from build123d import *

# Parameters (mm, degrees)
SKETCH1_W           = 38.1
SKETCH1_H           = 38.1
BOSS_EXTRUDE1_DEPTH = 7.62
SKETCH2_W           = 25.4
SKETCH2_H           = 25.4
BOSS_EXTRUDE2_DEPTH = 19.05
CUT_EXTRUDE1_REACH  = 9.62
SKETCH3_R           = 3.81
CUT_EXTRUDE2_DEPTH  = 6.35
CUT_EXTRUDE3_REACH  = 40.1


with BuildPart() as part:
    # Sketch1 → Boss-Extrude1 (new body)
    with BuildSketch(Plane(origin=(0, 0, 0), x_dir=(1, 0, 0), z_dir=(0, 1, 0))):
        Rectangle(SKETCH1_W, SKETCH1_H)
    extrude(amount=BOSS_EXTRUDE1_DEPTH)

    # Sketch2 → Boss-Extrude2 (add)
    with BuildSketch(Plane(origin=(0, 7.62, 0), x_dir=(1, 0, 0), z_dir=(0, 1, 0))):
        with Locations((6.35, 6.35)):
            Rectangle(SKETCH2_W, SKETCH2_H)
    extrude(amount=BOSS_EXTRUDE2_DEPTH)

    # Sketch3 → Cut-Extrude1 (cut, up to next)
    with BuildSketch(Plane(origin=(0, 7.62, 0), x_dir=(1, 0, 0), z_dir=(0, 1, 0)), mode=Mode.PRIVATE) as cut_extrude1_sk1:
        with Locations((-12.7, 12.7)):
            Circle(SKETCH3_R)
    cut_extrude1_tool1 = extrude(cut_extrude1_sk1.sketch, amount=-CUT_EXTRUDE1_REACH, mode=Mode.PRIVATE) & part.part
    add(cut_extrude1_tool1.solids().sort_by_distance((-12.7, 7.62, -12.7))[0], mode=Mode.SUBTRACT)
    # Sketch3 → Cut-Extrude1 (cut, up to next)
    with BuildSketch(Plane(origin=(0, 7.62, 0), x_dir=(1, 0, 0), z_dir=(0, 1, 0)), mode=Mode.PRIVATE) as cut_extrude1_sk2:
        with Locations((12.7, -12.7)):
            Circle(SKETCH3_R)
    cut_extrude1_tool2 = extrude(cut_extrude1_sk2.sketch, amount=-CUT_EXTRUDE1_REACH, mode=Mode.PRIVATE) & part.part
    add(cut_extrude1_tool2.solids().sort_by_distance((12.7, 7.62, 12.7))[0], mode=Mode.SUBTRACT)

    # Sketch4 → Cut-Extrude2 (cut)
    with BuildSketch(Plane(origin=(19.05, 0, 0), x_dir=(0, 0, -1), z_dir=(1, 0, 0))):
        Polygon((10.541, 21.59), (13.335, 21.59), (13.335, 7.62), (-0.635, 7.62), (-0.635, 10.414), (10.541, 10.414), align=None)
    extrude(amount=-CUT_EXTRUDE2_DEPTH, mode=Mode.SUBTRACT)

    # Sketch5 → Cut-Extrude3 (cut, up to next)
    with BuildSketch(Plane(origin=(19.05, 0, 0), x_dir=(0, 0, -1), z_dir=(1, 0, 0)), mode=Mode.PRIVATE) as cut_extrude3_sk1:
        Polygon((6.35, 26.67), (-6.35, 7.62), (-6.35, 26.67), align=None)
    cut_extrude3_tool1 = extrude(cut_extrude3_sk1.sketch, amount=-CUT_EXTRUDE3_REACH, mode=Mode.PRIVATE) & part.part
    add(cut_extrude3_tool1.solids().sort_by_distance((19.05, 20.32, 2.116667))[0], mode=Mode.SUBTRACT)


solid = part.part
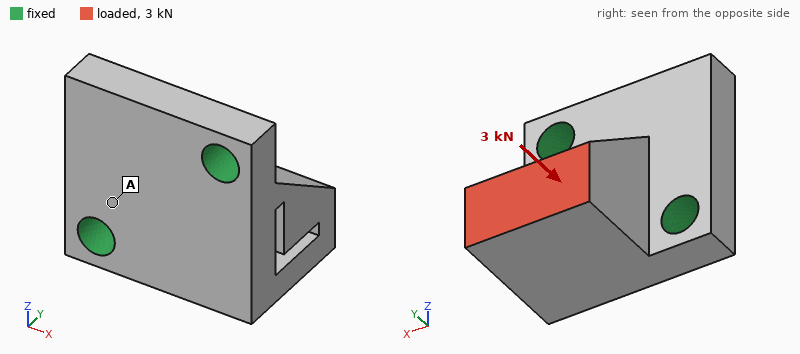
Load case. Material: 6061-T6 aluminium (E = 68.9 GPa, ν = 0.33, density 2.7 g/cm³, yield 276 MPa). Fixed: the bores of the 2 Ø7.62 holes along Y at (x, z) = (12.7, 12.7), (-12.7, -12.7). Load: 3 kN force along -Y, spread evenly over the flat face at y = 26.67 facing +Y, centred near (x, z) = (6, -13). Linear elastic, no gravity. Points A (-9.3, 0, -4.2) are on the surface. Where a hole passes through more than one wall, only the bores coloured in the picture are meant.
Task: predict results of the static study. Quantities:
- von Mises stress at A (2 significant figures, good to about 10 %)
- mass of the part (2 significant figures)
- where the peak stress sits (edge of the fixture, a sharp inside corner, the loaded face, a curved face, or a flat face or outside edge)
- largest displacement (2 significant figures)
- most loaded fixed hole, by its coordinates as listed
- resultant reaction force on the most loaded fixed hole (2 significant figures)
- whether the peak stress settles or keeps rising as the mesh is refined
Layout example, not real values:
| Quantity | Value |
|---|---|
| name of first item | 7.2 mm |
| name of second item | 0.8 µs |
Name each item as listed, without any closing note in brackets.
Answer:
| Quantity | Value |
|---|---|
| von Mises stress at A | 23 MPa |
| mass of the part | 52 g |
| where the peak stress sits | edge of the fixture |
| largest displacement | 73 µm |
| most loaded fixed hole, by its coordinates as listed | (-12.7, -12.7) |
| resultant reaction force on the most loaded fixed hole | 2.0 kN |
| whether the peak stress settles or keeps rising as the mesh is refined | keeps rising |
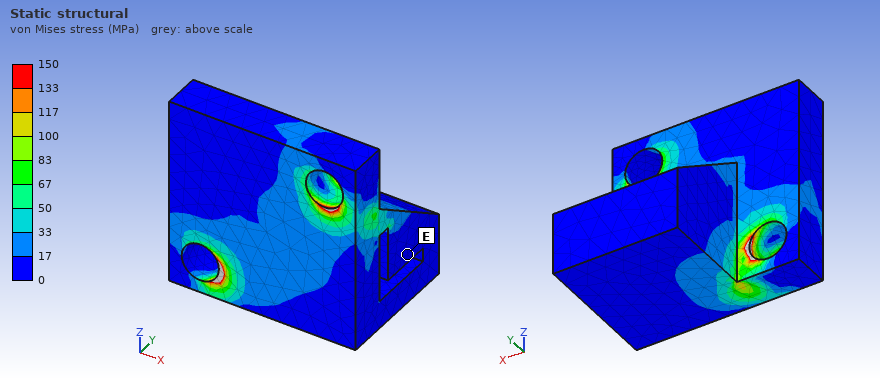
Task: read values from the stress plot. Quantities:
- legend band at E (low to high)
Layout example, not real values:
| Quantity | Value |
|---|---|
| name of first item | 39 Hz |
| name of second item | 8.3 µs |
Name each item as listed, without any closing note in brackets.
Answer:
| Quantity | Value |
|---|---|
| legend band at E | 0 to 17 MPa |
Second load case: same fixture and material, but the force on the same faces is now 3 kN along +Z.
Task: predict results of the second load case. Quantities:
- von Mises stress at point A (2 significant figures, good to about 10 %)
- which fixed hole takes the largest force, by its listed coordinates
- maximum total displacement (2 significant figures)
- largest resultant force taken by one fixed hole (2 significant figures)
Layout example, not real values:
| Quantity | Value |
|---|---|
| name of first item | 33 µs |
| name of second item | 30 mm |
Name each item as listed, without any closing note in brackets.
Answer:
| Quantity | Value |
|---|---|
| von Mises stress at point A | 25 MPa |
| which fixed hole takes the largest force, by its listed coordinates | (12.7, 12.7) |
| maximum total displacement | 0.10 mm |
| largest resultant force taken by one fixed hole | 2.4 kN |
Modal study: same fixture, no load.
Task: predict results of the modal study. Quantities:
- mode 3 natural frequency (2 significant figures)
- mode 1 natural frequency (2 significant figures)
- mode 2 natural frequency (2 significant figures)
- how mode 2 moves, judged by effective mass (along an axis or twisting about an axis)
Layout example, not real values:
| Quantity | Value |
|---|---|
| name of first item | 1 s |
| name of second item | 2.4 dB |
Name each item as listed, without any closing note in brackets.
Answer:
| Quantity | Value |
|---|---|
| mode 3 natural frequency | 18 kHz |
| mode 1 natural frequency | 6800 Hz |
| mode 2 natural frequency | 15 kHz |
| how mode 2 moves, judged by effective mass | along Y |
